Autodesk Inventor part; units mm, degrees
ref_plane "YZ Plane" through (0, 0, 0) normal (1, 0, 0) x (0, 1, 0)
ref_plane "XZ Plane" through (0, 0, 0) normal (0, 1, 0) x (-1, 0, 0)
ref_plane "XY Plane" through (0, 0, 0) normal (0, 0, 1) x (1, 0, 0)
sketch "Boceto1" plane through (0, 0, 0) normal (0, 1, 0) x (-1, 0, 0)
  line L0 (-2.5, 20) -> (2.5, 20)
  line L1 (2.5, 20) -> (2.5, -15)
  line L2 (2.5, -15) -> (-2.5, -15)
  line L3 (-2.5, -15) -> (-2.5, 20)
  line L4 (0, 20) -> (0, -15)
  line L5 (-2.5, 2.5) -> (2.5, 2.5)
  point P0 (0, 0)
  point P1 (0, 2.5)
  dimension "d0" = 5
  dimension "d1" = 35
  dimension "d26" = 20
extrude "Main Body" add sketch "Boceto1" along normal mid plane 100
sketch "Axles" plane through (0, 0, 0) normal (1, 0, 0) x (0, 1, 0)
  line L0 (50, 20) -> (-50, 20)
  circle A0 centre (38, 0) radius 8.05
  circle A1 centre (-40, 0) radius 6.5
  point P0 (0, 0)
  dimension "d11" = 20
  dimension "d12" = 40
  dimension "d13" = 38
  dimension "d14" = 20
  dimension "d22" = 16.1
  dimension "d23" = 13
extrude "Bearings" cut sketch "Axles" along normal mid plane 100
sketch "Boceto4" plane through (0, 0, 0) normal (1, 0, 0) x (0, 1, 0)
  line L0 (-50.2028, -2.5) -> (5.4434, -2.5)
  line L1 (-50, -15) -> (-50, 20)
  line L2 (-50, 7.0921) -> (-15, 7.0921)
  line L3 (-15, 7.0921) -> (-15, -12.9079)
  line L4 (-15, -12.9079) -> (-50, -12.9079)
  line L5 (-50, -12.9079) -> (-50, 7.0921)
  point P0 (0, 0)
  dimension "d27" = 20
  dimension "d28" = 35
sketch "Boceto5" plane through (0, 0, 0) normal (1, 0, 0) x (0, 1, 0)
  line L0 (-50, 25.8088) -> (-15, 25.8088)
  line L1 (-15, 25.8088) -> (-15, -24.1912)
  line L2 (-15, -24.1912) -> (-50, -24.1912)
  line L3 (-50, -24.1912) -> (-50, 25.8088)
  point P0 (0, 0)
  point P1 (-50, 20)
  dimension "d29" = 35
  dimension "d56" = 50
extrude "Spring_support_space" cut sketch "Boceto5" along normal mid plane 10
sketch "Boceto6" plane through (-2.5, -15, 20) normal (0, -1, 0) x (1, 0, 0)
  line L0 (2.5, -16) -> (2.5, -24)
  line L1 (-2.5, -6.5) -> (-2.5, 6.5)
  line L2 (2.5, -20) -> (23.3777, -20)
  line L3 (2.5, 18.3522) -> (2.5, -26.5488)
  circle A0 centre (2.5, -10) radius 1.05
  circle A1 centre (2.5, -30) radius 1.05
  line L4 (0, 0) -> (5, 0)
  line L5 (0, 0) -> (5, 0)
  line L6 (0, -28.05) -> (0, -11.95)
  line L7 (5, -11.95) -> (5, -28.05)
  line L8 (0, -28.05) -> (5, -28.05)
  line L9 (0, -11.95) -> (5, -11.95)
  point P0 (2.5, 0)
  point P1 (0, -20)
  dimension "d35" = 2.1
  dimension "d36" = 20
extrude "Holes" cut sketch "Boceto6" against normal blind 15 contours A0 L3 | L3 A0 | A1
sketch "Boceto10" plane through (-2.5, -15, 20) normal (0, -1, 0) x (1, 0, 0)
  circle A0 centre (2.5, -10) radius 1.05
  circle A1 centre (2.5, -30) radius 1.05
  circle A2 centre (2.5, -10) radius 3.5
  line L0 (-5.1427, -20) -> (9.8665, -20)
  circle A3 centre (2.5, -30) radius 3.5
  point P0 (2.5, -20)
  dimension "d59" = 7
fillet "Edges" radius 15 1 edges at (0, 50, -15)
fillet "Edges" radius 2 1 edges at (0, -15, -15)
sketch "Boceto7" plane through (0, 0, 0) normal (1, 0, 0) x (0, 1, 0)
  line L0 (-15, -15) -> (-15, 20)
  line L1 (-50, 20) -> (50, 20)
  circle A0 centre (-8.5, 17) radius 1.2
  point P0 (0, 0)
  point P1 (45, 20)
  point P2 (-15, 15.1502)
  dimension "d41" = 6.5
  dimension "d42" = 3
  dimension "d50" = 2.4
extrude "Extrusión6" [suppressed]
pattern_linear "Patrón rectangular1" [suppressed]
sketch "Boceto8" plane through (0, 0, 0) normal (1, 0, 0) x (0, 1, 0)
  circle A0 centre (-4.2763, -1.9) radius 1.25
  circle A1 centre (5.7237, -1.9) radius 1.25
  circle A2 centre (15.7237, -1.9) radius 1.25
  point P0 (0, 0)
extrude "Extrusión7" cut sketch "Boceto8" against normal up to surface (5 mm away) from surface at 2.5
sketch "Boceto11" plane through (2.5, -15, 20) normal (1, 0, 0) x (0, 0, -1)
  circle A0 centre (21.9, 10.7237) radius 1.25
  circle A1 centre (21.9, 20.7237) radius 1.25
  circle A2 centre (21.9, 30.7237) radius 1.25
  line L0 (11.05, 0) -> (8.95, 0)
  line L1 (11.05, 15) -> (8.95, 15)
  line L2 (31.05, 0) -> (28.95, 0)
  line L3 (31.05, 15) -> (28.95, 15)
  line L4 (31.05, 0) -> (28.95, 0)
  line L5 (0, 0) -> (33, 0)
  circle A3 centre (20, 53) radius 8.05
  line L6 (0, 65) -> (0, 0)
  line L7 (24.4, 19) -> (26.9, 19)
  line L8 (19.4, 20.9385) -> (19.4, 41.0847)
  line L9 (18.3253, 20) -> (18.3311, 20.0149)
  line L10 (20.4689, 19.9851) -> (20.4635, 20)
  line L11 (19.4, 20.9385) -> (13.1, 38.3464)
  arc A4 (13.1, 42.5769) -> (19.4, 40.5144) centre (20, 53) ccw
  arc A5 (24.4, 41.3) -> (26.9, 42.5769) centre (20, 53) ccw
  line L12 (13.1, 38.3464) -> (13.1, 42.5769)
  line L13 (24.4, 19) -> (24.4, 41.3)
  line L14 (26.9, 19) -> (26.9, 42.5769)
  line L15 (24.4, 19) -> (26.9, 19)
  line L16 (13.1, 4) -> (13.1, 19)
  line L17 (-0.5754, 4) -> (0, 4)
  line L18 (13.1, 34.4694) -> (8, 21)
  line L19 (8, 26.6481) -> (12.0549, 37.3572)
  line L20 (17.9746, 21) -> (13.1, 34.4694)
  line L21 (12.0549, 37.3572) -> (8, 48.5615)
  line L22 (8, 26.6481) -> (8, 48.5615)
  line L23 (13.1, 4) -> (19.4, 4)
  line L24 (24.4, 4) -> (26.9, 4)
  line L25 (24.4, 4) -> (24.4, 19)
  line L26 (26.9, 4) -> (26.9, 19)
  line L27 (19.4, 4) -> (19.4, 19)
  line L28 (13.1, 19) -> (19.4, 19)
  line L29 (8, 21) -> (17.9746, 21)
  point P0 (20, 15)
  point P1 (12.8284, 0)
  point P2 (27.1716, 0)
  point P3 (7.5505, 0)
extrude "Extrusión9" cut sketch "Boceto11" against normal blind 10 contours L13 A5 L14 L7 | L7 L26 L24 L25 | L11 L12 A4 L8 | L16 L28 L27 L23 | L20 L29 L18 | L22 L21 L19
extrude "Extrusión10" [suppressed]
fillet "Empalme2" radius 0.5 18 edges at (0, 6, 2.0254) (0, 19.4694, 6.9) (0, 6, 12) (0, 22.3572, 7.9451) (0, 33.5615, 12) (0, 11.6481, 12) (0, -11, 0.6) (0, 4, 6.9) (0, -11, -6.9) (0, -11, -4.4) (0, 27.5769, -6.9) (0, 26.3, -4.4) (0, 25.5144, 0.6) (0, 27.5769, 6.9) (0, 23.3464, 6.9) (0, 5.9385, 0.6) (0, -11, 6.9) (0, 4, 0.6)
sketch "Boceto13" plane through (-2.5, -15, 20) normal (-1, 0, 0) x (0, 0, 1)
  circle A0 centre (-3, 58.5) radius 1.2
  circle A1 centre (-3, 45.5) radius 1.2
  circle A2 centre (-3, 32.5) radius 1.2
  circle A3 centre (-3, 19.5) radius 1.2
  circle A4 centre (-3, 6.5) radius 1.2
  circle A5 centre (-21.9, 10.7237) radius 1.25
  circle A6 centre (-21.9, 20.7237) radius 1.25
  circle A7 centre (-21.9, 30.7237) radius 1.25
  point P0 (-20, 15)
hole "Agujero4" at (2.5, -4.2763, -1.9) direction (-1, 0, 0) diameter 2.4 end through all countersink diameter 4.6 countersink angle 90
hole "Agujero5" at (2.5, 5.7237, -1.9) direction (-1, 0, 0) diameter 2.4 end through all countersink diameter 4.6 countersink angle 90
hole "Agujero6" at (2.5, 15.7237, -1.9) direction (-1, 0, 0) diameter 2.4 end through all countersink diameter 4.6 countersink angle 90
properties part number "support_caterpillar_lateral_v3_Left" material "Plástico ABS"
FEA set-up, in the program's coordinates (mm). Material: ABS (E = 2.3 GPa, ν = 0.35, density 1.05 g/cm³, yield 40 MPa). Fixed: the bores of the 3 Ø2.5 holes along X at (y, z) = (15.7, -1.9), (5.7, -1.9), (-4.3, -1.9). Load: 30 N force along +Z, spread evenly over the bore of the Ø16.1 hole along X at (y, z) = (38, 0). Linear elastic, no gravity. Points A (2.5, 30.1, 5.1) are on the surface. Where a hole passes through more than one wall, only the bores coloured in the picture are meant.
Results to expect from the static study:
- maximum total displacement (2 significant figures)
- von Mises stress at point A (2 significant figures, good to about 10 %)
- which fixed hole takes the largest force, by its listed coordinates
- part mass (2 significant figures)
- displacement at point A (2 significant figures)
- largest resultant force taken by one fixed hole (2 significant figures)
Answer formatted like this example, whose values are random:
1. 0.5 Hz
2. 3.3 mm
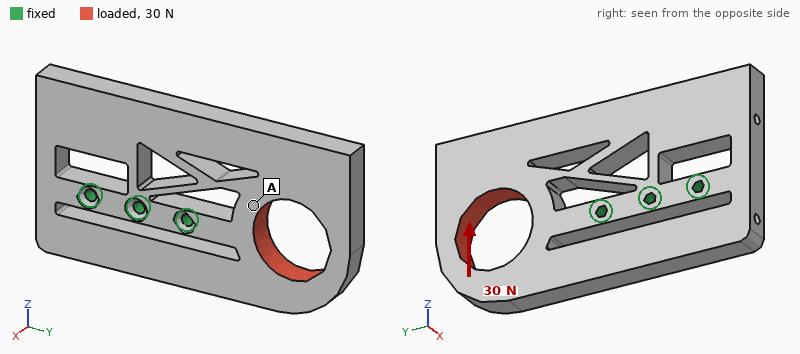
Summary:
1. 0.23 mm
2. 1.7 MPa
3. (15.7, -1.9)
4. 8.5 g
5. 0.11 mm
6. 44 N
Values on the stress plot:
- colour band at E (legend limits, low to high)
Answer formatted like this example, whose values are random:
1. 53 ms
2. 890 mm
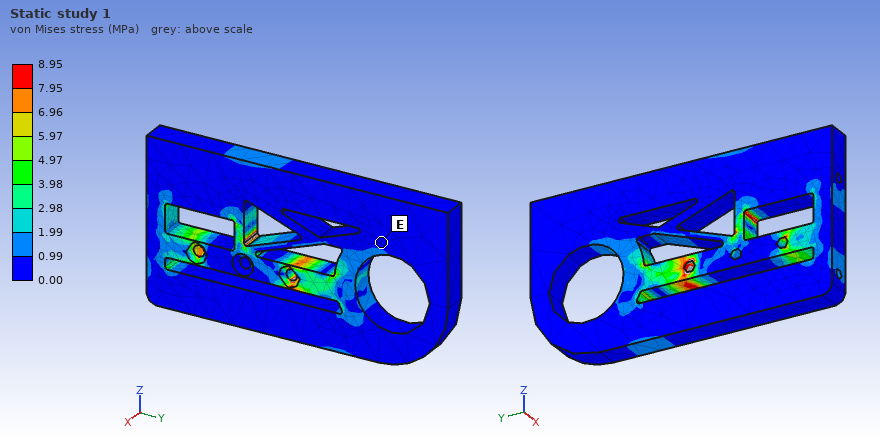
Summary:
1. 0.00 to 0.99 MPa
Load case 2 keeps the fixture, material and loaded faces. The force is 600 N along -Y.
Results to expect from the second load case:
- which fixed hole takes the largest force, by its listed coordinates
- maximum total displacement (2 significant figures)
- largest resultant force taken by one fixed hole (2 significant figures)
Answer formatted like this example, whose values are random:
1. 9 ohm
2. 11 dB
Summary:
1. (15.7, -1.9)
2. 0.31 mm
3. 340 N
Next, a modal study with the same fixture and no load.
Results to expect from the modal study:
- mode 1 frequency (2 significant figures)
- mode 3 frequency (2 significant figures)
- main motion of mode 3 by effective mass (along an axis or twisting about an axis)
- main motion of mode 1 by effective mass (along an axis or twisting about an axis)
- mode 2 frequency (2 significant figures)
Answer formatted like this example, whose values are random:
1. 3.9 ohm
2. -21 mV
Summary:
1. 590 Hz
2. 1000 Hz
3. along Z
4. along X
5. 870 Hz
